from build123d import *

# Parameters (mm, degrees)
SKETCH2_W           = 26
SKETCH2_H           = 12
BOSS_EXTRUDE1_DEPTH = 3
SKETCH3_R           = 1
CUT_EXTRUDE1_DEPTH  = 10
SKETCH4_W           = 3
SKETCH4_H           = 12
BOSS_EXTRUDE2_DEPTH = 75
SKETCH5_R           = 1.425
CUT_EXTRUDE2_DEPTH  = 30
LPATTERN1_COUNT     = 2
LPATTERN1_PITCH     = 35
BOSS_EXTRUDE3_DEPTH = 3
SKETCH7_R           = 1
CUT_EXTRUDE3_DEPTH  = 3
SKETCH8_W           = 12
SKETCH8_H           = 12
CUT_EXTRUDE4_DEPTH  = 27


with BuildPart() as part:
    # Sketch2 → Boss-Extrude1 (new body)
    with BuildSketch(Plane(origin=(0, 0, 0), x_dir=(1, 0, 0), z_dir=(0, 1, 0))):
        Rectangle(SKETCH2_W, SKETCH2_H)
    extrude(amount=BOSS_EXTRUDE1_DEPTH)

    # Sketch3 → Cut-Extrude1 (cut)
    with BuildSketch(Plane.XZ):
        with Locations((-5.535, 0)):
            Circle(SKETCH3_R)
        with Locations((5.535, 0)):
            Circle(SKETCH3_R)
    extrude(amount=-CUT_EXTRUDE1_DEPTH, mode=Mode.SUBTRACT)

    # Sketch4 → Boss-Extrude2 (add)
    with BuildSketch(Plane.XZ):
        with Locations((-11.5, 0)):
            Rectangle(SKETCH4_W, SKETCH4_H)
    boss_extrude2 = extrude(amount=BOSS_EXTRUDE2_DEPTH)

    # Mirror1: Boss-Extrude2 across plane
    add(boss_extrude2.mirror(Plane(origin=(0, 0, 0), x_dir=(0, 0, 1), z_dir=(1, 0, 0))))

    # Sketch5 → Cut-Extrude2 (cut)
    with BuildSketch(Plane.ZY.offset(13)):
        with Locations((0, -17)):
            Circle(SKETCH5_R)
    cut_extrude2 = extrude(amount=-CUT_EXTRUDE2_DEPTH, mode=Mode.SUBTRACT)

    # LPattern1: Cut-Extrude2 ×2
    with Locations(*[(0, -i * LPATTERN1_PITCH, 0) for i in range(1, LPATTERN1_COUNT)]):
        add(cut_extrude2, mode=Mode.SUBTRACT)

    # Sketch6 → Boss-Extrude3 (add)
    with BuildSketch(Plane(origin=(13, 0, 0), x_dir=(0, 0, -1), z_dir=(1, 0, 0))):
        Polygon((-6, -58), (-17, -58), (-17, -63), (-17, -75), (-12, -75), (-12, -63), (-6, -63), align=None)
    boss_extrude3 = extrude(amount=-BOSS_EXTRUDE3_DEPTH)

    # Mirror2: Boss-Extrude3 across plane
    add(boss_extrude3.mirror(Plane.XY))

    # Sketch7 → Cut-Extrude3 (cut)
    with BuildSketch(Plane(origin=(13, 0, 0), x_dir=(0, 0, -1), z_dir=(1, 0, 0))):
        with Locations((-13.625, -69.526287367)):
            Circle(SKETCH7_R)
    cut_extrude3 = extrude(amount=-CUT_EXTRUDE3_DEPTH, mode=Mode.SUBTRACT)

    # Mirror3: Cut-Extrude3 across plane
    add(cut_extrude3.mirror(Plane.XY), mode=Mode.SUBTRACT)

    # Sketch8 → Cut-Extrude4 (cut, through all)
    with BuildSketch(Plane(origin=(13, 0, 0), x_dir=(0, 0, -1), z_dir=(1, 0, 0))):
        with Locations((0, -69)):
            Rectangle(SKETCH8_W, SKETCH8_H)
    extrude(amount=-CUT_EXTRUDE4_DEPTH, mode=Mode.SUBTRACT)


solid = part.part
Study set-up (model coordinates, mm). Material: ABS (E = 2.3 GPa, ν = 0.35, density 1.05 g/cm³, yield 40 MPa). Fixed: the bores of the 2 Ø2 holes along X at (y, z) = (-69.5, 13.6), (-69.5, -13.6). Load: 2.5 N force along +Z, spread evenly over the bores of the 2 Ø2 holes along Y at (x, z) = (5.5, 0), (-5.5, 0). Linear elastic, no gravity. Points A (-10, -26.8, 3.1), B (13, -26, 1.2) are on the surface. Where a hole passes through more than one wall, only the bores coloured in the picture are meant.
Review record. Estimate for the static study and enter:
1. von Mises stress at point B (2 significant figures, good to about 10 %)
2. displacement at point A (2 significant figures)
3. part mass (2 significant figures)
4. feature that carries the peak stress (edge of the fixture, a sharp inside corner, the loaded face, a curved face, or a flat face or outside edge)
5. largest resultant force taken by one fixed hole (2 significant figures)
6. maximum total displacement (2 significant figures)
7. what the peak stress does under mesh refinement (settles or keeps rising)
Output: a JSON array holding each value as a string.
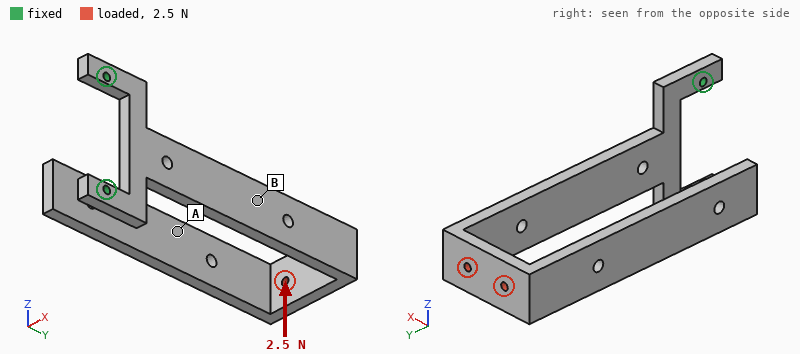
["1.4 MPa", "0.66 mm", "6.4 g", "a sharp inside corner", "6.8 N", "0.92 mm", "keeps rising"]
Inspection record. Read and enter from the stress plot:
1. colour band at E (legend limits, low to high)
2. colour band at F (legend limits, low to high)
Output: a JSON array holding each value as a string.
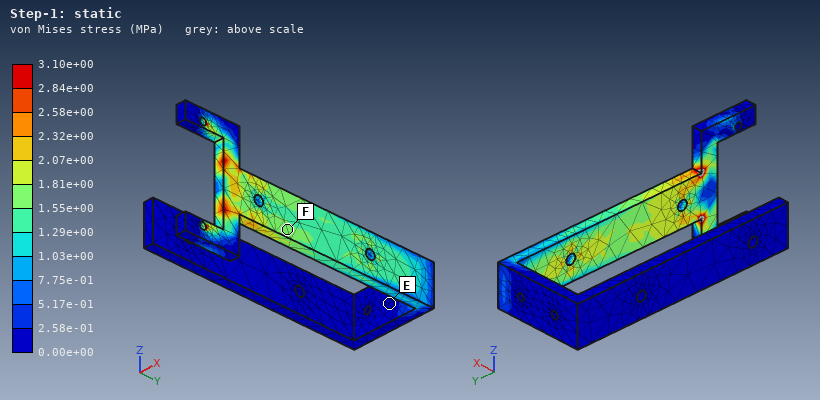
["0.00e+00 to 2.58e-01 MPa", "1.55e+00 to 1.81e+00 MPa"]
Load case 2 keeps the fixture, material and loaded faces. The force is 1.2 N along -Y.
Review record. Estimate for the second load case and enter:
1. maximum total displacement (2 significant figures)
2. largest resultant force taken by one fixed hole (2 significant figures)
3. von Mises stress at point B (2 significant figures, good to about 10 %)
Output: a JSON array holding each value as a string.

["0.89 mm", "0.70 N", "0.74 MPa"]
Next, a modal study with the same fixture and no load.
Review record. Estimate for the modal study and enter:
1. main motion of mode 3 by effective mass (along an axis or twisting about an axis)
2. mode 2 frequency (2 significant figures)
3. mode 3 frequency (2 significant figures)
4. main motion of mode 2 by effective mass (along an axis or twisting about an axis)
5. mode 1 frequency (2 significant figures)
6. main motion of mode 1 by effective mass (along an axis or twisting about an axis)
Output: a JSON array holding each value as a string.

["along Z", "86 Hz", "110 Hz", "along X", "59 Hz", "along X"]
